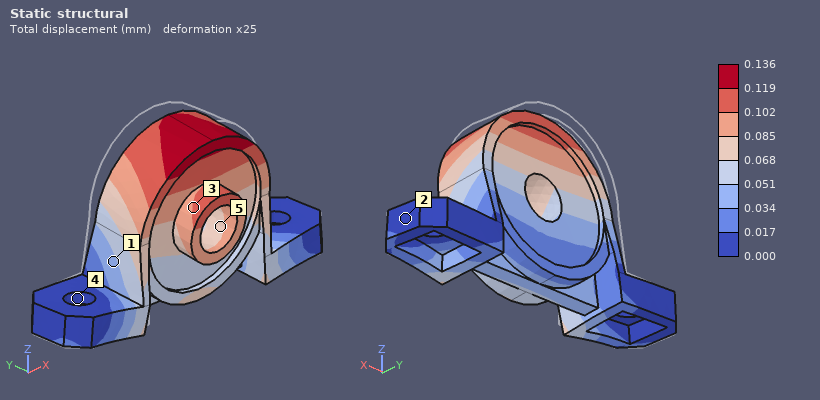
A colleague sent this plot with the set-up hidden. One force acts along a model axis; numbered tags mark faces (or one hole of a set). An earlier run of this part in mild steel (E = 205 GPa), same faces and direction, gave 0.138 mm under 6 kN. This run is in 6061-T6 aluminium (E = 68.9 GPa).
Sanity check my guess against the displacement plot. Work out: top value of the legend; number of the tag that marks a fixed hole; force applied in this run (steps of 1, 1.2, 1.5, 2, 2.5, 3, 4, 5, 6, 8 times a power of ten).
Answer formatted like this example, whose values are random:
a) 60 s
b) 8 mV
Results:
a) 0.136 mm
b) 4
c) 2 kN
